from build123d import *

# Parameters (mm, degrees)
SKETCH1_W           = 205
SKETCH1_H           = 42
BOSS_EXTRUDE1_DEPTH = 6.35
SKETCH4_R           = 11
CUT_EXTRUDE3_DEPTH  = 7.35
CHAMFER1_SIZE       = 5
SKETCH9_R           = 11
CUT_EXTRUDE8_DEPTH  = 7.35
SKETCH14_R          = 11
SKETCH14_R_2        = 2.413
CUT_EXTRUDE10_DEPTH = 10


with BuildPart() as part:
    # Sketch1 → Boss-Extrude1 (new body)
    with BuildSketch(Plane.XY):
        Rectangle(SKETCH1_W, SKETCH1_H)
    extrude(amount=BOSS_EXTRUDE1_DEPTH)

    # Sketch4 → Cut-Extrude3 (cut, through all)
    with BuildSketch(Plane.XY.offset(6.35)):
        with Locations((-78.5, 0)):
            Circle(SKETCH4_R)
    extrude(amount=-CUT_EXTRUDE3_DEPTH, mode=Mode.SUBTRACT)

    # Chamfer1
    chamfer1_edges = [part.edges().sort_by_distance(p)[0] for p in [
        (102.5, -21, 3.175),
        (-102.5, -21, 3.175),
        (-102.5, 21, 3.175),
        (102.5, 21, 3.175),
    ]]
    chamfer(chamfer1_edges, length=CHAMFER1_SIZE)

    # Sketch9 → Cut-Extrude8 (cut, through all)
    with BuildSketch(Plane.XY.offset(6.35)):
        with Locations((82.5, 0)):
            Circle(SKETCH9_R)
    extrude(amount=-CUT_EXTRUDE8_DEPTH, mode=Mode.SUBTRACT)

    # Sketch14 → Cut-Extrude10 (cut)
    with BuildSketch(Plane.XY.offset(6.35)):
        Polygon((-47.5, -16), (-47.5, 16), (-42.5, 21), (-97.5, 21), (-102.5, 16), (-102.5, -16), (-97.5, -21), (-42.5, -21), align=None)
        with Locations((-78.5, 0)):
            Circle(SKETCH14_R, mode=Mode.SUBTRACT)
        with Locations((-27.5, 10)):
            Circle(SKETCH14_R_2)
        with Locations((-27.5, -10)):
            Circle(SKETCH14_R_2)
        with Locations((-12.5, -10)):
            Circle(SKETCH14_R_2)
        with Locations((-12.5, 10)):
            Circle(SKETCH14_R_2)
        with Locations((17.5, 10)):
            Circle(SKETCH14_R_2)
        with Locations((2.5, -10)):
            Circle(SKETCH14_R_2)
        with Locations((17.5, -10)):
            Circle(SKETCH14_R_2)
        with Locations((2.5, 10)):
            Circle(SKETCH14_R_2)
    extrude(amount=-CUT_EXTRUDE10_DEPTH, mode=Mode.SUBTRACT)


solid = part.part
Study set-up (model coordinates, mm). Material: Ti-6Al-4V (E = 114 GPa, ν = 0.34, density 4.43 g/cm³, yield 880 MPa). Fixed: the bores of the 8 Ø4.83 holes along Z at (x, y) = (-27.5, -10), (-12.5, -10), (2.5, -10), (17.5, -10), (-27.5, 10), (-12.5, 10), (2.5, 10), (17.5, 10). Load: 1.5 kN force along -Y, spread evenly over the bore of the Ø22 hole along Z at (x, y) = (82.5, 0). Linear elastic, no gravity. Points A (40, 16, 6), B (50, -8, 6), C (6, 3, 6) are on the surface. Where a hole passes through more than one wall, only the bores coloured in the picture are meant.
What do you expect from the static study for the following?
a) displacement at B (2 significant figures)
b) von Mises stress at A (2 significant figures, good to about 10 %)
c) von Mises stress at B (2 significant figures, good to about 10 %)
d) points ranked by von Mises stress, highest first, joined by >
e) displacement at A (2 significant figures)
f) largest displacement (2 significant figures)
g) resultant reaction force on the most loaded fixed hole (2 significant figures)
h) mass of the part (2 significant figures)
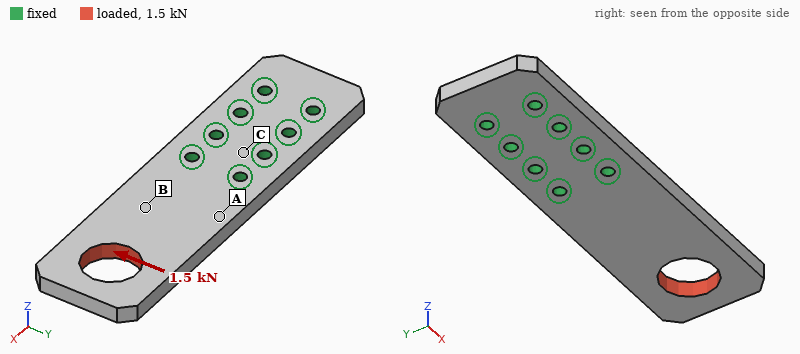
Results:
19 µm
27 MPa
16 MPa
A > B > C
14 µm
74 µm
3.0 kN
160 g
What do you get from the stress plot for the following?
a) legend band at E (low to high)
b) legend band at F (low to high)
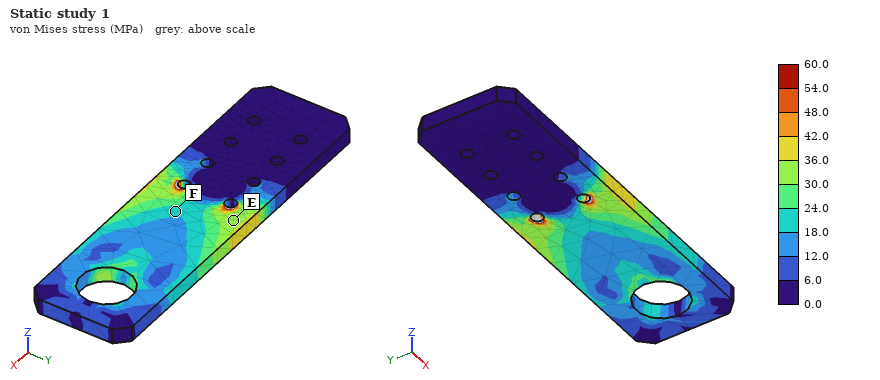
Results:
30.0 to 36.0 MPa
18.0 to 24.0 MPa
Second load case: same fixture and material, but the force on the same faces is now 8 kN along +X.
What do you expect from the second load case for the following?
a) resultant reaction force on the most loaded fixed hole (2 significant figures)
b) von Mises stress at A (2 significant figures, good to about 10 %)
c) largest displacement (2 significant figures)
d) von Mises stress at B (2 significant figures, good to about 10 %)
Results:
3.3 kN
30 MPa
33 µm
28 MPa
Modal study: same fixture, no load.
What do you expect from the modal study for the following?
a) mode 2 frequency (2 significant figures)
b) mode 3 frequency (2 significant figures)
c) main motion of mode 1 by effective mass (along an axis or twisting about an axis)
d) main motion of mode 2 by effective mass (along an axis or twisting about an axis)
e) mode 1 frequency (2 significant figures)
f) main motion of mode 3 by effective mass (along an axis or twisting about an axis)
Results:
2900 Hz
4000 Hz
along Z
twisting about X
830 Hz
along Y
